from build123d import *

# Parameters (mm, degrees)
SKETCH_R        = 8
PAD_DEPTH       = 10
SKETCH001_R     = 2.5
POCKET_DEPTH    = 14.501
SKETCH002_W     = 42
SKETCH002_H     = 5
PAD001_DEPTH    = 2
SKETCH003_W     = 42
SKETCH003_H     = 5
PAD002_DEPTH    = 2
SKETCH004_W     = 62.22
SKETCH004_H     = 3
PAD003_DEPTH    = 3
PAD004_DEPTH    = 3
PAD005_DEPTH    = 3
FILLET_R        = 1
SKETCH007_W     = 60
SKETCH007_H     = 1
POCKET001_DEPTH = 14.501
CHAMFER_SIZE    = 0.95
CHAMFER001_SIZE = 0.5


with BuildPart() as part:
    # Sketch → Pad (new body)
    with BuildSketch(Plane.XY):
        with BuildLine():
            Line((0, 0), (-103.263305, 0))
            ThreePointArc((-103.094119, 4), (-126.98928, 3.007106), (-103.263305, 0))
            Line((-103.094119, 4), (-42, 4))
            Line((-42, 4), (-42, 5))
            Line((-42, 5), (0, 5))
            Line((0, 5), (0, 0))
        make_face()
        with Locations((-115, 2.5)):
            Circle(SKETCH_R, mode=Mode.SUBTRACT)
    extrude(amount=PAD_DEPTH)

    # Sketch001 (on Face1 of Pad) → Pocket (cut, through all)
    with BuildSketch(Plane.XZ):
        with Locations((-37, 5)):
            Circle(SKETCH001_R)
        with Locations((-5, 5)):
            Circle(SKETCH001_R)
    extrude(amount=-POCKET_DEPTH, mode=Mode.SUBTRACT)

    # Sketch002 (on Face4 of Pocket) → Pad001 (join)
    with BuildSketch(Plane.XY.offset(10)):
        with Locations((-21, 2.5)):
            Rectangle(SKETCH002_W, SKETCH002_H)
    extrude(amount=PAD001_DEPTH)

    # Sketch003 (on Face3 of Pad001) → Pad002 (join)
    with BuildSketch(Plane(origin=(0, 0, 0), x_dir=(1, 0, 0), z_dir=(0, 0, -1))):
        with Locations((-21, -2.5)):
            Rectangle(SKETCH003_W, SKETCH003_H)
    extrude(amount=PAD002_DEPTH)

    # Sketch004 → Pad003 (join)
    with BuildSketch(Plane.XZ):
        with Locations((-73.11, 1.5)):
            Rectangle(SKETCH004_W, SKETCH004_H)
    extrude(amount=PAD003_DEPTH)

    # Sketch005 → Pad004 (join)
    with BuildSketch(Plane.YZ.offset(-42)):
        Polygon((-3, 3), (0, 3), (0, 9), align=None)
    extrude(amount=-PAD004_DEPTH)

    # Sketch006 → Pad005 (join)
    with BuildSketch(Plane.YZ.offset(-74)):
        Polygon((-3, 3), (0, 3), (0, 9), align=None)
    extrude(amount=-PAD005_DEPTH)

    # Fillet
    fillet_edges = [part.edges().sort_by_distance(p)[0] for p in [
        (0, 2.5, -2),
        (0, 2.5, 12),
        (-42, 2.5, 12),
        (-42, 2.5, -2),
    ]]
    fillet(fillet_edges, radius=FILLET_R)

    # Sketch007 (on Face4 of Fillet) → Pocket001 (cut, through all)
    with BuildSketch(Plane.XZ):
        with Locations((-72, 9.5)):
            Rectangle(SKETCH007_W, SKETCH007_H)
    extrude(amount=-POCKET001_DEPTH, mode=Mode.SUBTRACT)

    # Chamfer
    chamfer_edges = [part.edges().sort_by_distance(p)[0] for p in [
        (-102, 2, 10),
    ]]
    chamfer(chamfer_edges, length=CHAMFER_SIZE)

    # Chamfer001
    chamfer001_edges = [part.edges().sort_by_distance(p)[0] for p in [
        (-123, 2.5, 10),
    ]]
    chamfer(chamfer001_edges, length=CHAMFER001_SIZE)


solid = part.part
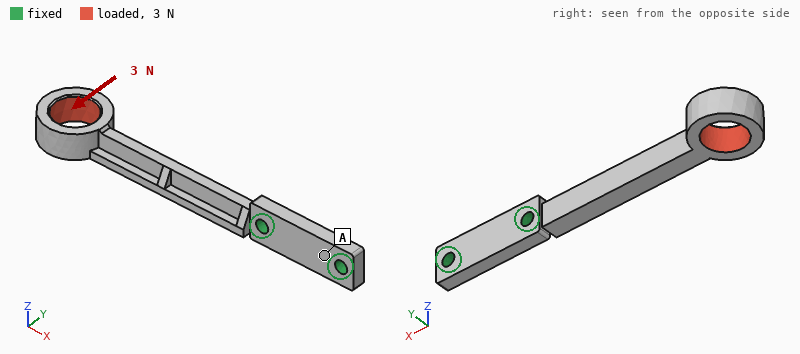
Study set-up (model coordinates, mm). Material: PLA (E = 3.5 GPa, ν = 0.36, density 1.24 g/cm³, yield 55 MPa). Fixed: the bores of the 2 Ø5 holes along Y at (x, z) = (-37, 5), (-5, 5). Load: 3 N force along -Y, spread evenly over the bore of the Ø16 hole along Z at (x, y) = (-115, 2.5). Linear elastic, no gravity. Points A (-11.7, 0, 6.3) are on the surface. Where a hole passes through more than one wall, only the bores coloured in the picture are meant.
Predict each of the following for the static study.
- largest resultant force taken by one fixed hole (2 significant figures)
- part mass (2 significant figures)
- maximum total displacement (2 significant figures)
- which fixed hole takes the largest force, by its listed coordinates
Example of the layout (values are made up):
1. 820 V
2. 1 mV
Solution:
1. 3.2 N
2. 10.0 g
3. 1.5 mm
4. (-37, 5)
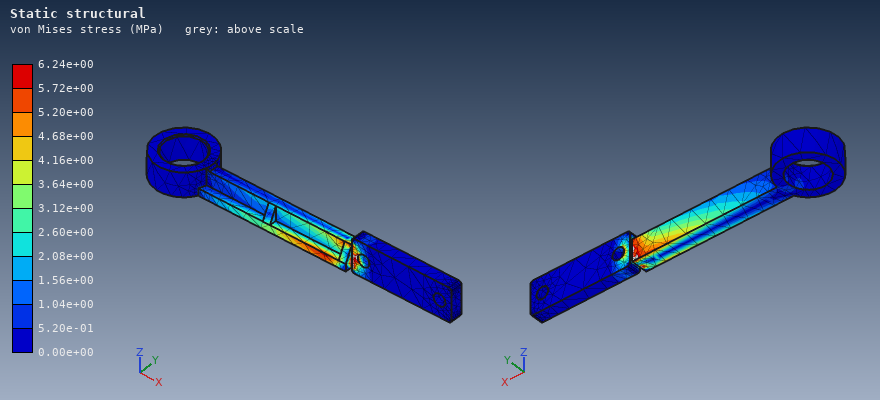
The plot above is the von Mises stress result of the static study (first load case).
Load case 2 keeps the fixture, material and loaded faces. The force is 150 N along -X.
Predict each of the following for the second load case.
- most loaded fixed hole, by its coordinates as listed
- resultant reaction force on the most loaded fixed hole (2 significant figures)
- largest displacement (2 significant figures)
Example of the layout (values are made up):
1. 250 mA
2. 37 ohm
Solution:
1. (-37, 5)
2. 140 N
3. 1.3 mm
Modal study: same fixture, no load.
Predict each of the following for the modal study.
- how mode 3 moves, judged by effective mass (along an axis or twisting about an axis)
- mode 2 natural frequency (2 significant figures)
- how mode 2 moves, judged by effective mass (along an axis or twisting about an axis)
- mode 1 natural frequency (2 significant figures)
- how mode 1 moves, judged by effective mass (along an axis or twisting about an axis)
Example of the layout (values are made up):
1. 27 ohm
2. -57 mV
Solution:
1. twisting about X
2. 220 Hz
3. along Z
4. 130 Hz
5. along Y
